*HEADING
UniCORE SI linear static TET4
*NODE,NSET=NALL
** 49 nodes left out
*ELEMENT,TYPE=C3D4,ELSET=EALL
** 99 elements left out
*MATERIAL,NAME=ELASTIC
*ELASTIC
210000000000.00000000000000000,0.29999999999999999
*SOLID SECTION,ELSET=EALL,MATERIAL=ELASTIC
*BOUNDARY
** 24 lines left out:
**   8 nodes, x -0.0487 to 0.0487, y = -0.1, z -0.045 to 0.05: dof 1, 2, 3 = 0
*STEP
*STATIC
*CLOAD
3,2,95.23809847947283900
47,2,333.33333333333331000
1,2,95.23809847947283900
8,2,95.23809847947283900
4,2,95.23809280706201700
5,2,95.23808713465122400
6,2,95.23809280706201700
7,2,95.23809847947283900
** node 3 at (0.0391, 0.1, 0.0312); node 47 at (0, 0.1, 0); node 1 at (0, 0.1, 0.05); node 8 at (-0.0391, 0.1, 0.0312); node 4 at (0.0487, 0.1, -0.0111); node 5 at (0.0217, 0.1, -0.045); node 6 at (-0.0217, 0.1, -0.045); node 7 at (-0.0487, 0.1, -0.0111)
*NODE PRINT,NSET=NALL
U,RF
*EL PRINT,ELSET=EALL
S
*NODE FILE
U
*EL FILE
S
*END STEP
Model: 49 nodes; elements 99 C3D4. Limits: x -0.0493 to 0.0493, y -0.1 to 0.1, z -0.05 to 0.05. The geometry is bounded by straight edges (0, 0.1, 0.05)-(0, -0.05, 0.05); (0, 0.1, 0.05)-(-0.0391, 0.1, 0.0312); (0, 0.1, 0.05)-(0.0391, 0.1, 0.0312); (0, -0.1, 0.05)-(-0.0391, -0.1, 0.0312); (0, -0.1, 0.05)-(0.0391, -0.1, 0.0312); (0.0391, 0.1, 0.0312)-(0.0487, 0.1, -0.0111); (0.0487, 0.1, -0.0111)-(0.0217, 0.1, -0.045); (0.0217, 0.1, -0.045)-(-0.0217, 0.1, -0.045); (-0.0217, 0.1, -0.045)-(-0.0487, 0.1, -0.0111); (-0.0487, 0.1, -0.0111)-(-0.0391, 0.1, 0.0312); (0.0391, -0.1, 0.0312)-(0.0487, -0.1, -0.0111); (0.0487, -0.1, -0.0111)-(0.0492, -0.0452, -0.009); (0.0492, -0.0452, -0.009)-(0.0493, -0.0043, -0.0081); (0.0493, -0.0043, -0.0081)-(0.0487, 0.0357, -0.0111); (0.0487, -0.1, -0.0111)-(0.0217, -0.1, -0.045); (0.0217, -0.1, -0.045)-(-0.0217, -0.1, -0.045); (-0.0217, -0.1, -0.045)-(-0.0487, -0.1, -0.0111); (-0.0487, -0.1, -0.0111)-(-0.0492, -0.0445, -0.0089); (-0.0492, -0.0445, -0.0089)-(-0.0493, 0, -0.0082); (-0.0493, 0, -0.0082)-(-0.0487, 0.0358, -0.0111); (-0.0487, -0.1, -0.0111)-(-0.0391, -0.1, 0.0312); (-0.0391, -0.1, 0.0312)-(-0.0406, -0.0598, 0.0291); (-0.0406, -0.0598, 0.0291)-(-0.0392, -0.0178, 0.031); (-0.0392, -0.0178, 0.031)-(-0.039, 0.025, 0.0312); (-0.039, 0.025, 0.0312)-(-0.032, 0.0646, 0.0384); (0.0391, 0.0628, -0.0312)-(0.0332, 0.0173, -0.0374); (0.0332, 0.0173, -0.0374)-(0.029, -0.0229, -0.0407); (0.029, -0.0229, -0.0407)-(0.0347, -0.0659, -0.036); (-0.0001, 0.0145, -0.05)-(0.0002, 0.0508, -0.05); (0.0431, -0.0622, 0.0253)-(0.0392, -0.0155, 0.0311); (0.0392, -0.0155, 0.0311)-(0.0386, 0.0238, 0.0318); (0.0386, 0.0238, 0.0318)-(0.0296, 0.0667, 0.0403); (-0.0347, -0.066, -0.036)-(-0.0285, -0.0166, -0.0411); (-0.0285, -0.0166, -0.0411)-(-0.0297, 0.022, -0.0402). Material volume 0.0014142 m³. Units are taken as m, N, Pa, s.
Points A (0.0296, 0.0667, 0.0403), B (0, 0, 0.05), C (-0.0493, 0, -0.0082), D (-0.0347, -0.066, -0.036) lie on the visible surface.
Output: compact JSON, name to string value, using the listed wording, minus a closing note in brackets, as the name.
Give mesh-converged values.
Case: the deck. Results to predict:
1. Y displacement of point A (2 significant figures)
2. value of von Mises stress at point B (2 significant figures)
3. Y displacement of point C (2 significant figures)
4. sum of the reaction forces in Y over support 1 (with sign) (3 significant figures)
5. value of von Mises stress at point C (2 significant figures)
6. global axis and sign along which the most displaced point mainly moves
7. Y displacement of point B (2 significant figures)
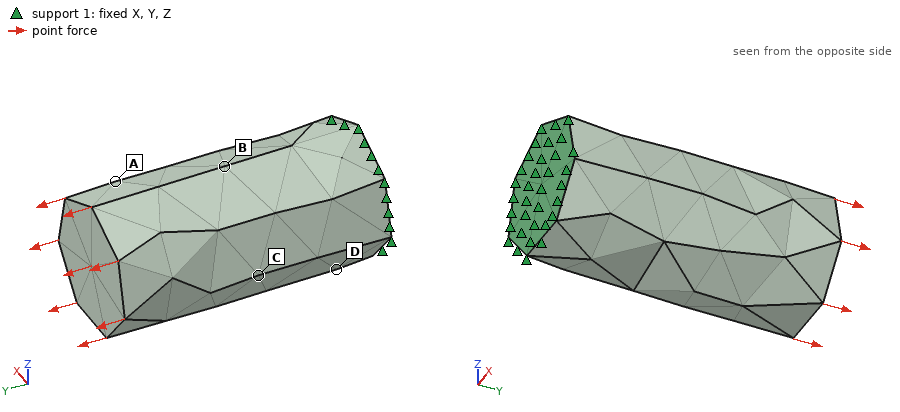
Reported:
{"Y displacement of point A": "1.1e-07 m", "value of von Mises stress at point B": "1.5e+05 Pa", "Y displacement of point C": "6.6e-08 m", "sum of the reaction forces in Y over support 1 (with sign)": "-1000 N", "value of von Mises stress at point C": "1.4e+05 Pa", "global axis and sign along which the most displaced point mainly moves": "+Y", "Y displacement of point B": "6.7e-08 m"}
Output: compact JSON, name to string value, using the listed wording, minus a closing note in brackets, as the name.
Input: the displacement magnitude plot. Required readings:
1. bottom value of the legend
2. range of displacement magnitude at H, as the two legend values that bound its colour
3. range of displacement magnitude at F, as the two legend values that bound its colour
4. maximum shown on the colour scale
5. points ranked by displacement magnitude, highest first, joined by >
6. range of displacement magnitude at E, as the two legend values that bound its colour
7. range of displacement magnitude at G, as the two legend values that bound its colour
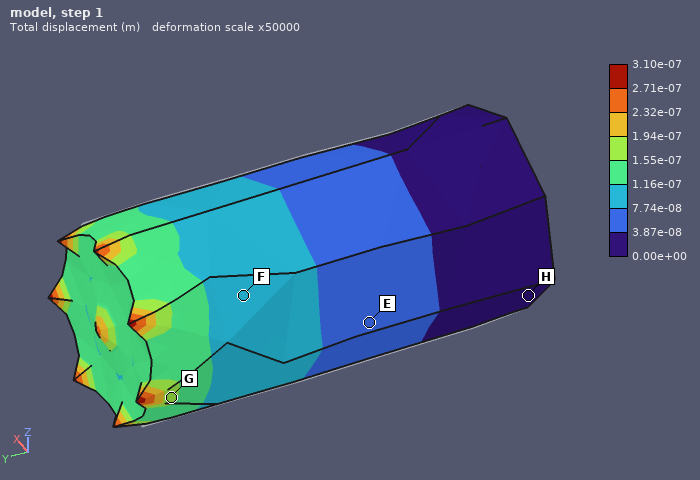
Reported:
{"bottom value of the legend": "0.00e+00 m", "range of displacement magnitude at H, as the two legend values that bound its colour": "0.00e+00 to 3.87e-08 m", "range of displacement magnitude at F, as the two legend values that bound its colour": "7.74e-08 to 1.16e-07 m", "maximum shown on the colour scale": "3.10e-07 m", "points ranked by displacement magnitude, highest first, joined by >": "G > F > E > H", "range of displacement magnitude at E, as the two legend values that bound its colour": "3.87e-08 to 7.74e-08 m", "range of displacement magnitude at G, as the two legend values that bound its colour": "1.55e-07 to 1.94e-07 m"}
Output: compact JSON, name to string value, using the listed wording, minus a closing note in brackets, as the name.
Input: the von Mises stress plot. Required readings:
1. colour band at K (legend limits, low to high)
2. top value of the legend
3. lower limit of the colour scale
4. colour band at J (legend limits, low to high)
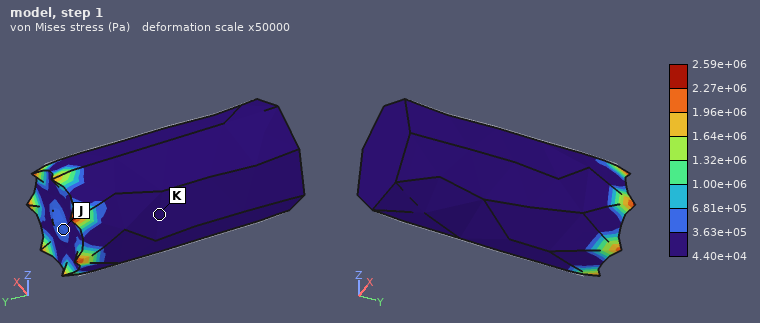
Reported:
{"colour band at K": "4.40e+04 to 3.63e+05 Pa", "top value of the legend": "2.59e+06 Pa", "lower limit of the colour scale": "4.40e+04 Pa", "colour band at J": "3.63e+05 to 6.81e+05 Pa"}
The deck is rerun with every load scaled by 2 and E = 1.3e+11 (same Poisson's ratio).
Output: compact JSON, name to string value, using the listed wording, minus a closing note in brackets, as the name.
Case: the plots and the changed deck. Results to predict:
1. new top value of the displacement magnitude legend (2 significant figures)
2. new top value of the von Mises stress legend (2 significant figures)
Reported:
{"new top value of the displacement magnitude legend": "1.0e-06 m", "new top value of the von Mises stress legend": "5.2e+06 Pa"}
